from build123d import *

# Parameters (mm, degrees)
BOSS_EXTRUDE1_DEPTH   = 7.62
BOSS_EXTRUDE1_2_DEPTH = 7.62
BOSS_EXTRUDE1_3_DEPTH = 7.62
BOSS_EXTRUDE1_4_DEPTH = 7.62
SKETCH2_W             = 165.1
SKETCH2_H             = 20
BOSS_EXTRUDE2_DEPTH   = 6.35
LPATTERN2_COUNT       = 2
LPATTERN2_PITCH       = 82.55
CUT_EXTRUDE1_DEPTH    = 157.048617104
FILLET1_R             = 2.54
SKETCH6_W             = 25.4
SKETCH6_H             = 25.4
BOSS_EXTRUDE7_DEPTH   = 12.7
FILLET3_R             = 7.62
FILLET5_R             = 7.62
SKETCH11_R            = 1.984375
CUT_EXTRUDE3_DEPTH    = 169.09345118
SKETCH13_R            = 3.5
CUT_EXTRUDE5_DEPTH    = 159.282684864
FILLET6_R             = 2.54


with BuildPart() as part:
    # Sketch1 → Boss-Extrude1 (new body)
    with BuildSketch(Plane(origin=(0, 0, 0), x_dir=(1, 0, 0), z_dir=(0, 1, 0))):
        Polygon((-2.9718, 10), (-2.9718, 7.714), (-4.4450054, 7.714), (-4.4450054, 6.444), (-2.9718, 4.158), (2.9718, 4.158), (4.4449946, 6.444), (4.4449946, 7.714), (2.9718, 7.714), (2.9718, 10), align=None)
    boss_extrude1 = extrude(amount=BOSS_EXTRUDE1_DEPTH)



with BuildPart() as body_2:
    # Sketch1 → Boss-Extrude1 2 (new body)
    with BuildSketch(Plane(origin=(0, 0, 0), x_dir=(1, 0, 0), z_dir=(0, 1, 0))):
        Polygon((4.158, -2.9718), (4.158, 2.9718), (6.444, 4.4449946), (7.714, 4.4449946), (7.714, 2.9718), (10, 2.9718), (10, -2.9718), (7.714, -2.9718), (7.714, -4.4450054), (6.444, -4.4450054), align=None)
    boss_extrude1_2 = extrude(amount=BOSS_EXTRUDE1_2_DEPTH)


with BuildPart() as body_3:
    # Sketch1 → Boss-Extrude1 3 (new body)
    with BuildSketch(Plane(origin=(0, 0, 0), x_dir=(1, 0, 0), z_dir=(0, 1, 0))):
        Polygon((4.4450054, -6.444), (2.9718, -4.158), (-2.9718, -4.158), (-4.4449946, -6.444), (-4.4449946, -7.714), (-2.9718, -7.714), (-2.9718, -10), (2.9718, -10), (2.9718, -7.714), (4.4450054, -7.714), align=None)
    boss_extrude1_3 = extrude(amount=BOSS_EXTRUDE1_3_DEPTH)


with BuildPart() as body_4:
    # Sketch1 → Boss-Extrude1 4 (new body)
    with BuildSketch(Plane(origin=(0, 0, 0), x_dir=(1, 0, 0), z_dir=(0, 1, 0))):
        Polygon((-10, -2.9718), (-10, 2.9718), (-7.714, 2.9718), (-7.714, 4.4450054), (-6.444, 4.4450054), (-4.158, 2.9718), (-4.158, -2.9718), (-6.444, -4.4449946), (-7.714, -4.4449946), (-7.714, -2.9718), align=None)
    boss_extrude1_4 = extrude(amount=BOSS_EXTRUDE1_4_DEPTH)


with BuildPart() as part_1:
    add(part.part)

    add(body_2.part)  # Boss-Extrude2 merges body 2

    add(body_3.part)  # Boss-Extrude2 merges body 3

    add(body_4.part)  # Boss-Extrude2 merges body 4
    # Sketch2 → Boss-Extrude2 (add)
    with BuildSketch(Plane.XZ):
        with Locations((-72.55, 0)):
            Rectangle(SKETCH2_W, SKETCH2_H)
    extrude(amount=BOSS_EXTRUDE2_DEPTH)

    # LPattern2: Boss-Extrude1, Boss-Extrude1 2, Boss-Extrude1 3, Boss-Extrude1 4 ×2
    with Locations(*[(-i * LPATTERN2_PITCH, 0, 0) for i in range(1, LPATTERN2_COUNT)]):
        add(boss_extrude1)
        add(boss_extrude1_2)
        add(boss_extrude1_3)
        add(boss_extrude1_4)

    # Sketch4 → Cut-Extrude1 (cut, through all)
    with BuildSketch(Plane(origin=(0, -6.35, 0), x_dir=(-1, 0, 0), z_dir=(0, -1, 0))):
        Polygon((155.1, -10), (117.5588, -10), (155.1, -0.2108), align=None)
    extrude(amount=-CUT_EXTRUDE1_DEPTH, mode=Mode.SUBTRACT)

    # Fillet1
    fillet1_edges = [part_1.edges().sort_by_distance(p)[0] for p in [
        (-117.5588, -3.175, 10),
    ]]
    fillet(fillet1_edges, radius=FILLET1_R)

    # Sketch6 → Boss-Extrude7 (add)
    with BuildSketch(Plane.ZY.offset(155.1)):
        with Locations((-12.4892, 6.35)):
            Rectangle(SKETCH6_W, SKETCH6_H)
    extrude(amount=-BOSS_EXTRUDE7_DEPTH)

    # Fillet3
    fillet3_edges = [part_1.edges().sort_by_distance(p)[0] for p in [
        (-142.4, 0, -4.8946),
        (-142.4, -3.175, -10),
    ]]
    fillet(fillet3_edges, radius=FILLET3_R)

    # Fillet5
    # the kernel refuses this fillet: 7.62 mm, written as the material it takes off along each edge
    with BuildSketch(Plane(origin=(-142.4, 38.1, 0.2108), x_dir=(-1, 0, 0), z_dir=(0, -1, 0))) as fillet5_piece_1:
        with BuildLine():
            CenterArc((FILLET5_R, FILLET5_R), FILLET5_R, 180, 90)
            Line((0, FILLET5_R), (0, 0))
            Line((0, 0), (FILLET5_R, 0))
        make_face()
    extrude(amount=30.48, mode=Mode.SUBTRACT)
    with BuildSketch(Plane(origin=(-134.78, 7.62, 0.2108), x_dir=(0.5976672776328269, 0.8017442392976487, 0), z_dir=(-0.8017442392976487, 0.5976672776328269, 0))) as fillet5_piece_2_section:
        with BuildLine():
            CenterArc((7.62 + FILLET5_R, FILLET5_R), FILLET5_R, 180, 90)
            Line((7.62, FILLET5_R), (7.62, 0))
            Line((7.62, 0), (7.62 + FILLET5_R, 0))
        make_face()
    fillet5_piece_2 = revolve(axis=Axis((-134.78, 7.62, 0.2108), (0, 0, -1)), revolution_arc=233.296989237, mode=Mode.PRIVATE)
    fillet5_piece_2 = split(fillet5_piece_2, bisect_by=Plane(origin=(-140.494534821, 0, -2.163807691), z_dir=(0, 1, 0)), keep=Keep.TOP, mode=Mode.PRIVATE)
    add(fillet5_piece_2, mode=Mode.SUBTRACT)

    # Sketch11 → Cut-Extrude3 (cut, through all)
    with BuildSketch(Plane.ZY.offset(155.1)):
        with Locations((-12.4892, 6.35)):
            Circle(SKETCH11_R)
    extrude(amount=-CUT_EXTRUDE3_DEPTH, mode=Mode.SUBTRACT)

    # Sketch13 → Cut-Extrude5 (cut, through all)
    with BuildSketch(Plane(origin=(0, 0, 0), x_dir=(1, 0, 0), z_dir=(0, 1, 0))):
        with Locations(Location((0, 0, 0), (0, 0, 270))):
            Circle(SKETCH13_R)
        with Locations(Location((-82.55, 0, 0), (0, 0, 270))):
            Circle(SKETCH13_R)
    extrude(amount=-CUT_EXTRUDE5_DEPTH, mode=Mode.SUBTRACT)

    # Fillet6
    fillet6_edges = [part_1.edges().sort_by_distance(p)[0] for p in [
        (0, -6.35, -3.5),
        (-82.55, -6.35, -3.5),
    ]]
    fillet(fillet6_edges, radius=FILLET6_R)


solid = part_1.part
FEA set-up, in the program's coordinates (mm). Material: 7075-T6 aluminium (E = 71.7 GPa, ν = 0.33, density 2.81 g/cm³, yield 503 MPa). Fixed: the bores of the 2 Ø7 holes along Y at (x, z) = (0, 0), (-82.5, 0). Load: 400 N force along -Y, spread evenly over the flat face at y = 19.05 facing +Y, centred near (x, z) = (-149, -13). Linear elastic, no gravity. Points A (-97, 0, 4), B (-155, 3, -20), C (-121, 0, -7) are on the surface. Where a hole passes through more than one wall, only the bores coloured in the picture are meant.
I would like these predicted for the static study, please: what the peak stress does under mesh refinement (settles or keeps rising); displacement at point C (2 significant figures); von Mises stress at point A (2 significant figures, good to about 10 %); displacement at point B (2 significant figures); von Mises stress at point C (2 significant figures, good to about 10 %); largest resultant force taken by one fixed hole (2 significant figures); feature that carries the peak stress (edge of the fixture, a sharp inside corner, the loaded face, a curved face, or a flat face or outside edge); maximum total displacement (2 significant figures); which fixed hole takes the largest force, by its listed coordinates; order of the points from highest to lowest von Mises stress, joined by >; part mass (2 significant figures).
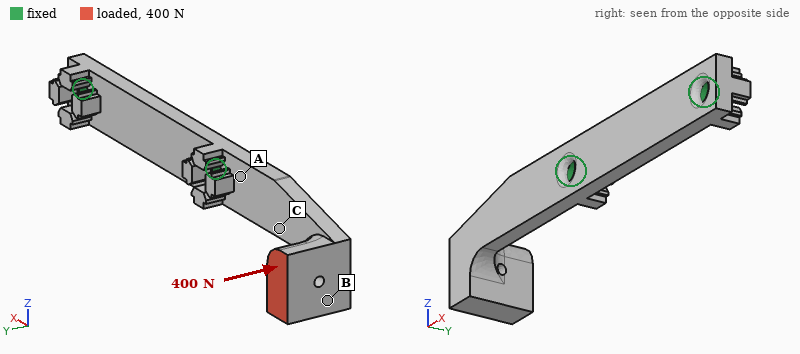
keeps rising
0.55 mm
150 MPa
1.7 mm
100 MPa
480 N
edge of the fixture
1.8 mm
(-82.5, 0)
A > C > B
81 g
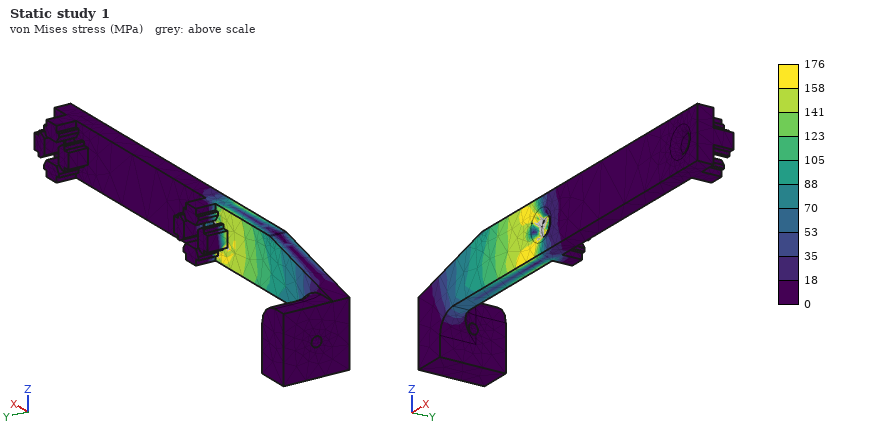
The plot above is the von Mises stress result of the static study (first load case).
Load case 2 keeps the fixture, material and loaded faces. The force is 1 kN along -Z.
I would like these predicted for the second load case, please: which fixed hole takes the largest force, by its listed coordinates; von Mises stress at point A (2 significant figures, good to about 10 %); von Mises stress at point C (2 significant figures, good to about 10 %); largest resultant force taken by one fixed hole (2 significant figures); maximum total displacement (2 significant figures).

(-82.5, 0)
180 MPa
170 MPa
1.3 kN
1.7 mm
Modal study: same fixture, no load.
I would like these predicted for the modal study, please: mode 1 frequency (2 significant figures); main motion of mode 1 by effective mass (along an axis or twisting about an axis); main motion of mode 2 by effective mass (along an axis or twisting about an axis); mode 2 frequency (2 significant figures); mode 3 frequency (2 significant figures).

520 Hz
along Y
along Z
1200 Hz
2400 Hz
